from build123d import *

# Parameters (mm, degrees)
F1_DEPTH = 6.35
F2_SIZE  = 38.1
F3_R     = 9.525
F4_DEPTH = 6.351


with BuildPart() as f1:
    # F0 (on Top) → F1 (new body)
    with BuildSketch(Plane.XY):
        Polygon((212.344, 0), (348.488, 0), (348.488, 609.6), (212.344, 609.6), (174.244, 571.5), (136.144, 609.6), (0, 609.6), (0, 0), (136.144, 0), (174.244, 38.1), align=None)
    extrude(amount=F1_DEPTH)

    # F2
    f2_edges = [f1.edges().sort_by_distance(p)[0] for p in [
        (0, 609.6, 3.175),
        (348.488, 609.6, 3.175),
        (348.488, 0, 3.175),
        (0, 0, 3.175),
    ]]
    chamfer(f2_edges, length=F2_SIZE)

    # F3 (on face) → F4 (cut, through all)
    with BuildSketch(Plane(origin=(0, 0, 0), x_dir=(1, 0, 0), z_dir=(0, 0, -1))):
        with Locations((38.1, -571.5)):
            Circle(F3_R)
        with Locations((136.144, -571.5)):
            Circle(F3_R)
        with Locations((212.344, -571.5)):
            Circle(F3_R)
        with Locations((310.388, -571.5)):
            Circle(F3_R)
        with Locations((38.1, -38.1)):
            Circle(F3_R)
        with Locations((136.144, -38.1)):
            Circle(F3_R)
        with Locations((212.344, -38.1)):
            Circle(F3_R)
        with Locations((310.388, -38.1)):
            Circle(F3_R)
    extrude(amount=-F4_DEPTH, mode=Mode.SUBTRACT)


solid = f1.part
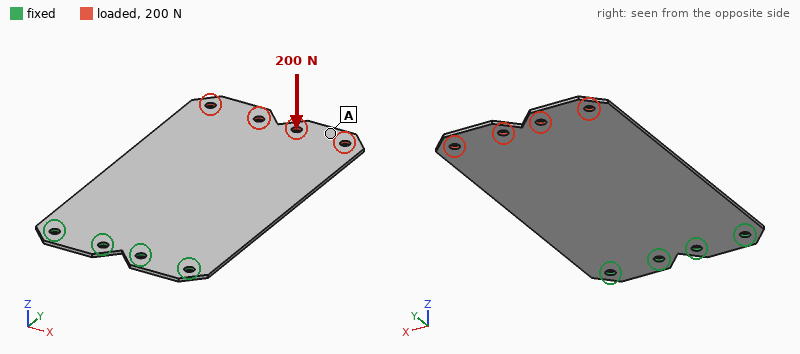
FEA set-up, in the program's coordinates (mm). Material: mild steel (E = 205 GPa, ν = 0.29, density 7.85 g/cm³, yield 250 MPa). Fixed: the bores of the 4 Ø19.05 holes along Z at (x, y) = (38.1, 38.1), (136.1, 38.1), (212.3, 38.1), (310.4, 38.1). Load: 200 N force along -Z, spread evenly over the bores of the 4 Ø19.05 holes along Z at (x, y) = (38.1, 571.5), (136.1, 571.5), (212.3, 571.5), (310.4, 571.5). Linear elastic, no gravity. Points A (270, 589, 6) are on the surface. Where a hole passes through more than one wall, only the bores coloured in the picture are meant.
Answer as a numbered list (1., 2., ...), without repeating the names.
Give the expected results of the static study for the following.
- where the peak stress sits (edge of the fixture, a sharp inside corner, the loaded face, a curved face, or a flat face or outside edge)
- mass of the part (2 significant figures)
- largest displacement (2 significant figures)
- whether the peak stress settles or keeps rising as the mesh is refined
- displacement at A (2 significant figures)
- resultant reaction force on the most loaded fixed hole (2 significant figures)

1. edge of the fixture
2. 10 kg
3. 7.0 mm
4. keeps rising
5. 6.6 mm
6. 120 N
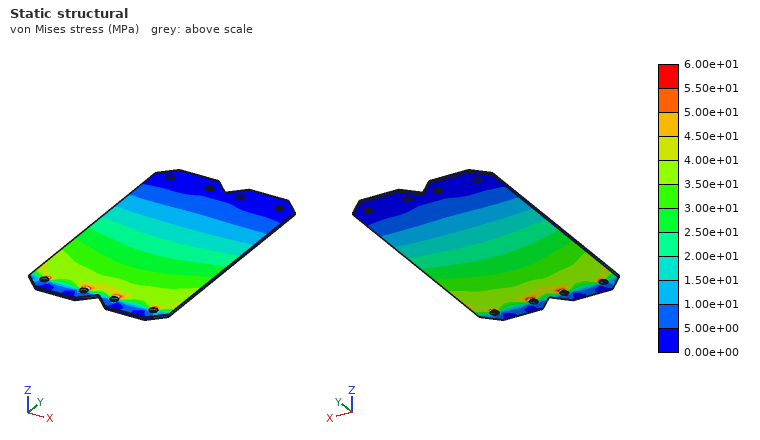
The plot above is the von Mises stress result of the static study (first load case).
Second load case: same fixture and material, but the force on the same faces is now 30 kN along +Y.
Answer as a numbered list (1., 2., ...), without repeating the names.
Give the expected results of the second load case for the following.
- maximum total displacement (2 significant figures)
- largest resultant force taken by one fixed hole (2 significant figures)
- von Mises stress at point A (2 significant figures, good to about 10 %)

1. 40 µm
2. 8.0 kN
3. 4.1 MPa
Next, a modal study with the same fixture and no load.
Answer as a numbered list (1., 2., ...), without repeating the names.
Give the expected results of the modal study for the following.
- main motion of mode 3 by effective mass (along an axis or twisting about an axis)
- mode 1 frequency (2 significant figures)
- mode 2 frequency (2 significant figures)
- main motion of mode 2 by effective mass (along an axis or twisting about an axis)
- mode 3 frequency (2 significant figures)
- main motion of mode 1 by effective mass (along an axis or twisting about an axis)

1. along Z
2. 17 Hz
3. 62 Hz
4. twisting about Y
5. 110 Hz
6. along Z
